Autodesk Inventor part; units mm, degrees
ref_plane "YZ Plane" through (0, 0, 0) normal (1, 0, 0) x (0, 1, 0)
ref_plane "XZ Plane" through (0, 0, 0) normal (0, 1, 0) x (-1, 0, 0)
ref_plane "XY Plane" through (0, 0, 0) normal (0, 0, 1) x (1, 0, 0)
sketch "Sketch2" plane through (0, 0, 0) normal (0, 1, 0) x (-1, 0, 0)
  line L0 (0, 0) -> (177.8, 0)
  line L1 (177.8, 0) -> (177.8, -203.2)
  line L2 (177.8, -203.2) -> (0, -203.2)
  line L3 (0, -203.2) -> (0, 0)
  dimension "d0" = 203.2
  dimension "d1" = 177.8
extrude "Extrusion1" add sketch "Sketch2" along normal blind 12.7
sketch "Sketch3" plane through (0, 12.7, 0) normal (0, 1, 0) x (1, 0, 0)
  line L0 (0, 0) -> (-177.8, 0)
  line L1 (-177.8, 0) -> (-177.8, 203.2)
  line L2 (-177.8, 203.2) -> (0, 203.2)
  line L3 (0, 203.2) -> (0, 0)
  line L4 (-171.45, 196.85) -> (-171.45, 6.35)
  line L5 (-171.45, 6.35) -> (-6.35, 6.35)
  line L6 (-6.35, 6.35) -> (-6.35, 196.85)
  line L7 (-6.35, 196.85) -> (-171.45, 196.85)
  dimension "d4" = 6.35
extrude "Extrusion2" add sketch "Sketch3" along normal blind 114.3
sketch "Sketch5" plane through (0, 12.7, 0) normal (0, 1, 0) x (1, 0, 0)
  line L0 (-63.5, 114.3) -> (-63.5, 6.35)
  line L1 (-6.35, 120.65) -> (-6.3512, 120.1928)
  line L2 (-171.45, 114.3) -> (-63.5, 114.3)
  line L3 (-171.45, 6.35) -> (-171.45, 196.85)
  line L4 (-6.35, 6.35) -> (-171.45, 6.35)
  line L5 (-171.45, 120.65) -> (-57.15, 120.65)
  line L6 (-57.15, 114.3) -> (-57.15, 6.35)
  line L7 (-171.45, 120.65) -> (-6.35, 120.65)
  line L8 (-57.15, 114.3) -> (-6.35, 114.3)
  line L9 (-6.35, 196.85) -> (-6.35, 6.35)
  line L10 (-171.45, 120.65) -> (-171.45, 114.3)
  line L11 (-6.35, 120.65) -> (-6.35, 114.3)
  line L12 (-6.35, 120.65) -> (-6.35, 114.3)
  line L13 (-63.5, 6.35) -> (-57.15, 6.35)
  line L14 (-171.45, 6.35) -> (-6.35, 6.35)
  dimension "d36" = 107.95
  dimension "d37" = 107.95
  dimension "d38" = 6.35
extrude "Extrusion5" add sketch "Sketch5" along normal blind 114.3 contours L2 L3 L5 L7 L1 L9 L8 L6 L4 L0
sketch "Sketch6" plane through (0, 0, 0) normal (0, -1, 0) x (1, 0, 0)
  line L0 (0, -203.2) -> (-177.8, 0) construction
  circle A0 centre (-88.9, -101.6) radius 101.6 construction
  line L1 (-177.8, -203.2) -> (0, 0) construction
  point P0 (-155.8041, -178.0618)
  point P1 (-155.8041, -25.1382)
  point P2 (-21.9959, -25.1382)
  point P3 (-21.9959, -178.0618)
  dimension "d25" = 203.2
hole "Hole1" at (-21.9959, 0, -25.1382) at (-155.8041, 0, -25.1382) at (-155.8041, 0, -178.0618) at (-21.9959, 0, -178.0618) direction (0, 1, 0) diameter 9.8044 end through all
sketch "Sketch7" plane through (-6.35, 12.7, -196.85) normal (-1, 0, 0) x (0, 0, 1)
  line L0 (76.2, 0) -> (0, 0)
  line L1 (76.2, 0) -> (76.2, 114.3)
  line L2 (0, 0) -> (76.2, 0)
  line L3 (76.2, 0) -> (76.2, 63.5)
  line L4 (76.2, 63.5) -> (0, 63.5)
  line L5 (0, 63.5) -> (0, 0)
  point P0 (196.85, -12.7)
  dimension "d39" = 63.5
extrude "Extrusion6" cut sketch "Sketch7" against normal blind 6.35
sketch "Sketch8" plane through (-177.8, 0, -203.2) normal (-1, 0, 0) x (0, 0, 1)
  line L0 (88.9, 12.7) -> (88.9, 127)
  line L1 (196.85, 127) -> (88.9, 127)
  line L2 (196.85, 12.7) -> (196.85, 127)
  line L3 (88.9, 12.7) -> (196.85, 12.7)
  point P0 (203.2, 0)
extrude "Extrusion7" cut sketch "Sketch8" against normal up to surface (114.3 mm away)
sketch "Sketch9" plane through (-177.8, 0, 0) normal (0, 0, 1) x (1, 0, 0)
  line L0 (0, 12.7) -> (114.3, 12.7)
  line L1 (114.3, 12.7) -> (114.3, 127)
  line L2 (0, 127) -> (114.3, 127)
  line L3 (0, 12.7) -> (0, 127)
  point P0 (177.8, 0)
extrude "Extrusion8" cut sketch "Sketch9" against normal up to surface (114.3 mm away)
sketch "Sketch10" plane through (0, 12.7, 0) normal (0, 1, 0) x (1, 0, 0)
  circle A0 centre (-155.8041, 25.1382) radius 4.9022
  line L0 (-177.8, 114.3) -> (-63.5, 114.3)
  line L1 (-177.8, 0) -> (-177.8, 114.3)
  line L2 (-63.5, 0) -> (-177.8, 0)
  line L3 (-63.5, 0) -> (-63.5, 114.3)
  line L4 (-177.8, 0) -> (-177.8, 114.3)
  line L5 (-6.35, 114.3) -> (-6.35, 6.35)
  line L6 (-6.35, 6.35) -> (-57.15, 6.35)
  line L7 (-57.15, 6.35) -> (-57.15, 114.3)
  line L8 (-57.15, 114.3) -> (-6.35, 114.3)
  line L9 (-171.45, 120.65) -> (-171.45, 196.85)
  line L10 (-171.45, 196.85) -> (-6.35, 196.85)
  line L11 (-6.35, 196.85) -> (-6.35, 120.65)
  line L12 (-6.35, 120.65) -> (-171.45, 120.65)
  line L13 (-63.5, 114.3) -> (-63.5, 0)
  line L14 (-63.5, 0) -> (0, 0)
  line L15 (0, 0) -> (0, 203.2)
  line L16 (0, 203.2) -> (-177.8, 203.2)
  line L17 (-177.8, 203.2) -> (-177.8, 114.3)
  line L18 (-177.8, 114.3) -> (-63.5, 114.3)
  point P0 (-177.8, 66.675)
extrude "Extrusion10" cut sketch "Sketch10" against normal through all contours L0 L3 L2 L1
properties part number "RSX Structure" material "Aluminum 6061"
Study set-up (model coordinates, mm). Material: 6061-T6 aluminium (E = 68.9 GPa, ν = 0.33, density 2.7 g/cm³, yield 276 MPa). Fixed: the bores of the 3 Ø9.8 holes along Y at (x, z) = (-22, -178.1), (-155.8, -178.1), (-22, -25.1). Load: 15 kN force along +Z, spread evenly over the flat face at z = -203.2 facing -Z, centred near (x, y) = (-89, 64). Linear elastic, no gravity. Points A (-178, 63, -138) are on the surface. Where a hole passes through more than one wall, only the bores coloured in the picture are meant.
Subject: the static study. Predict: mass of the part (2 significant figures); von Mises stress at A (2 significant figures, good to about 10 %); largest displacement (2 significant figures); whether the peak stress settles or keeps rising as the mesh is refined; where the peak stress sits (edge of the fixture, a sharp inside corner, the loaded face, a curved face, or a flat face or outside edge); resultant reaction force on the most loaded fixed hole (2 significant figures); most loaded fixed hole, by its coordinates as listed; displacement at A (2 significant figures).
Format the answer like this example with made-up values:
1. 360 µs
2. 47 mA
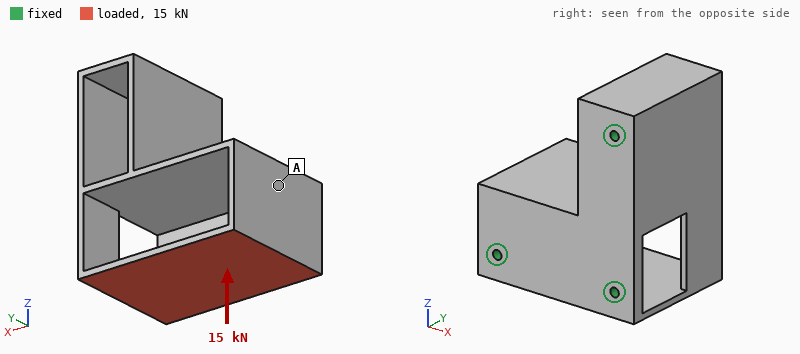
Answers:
1. 2.2 kg
2. 21 MPa
3. 1.8 mm
4. keeps rising
5. edge of the fixture
6. 7.6 kN
7. (-155.8, -178.1)
8. 0.36 mm
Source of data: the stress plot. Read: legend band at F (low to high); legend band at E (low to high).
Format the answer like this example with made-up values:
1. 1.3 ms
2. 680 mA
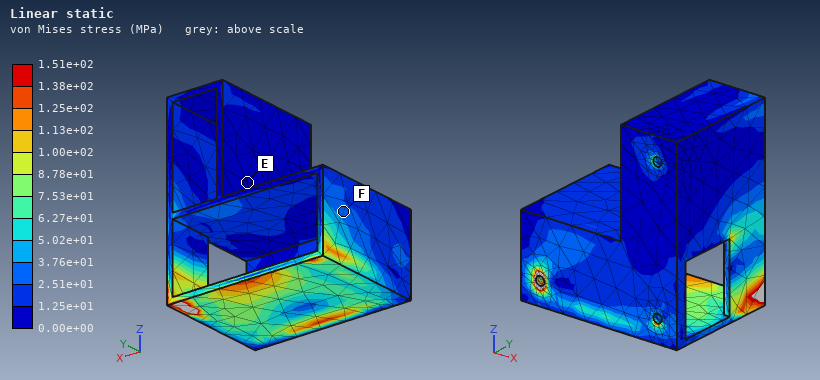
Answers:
1. 2.51e+01 to 3.76e+01 MPa
2. 0.00e+00 to 1.25e+01 MPa
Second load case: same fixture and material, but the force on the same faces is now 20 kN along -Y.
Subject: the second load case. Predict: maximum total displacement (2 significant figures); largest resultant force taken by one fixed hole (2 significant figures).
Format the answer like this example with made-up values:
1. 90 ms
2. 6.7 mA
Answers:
1. 0.38 mm
2. 11 kN
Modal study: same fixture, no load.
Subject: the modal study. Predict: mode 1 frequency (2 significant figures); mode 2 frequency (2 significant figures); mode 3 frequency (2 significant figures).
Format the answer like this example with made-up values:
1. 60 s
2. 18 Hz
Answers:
1. 790 Hz
2. 1100 Hz
3. 1300 Hz
